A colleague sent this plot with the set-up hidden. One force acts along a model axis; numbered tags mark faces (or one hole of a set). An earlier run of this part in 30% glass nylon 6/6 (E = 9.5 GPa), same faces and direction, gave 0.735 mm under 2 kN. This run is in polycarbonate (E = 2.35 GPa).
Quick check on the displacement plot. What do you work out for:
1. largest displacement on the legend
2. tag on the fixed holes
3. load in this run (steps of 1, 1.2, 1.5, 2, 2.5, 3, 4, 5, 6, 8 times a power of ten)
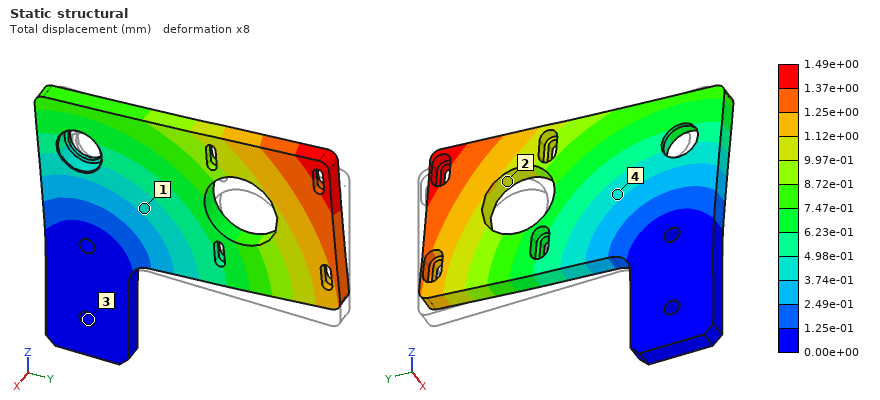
1.49e+00 mm
3
1 kN
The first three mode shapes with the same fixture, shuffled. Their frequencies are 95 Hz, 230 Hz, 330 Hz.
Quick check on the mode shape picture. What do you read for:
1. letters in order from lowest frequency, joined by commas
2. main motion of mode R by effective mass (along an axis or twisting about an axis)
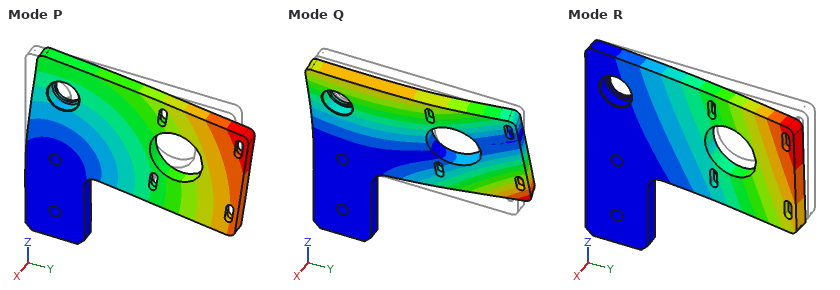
R, Q, P
along X
